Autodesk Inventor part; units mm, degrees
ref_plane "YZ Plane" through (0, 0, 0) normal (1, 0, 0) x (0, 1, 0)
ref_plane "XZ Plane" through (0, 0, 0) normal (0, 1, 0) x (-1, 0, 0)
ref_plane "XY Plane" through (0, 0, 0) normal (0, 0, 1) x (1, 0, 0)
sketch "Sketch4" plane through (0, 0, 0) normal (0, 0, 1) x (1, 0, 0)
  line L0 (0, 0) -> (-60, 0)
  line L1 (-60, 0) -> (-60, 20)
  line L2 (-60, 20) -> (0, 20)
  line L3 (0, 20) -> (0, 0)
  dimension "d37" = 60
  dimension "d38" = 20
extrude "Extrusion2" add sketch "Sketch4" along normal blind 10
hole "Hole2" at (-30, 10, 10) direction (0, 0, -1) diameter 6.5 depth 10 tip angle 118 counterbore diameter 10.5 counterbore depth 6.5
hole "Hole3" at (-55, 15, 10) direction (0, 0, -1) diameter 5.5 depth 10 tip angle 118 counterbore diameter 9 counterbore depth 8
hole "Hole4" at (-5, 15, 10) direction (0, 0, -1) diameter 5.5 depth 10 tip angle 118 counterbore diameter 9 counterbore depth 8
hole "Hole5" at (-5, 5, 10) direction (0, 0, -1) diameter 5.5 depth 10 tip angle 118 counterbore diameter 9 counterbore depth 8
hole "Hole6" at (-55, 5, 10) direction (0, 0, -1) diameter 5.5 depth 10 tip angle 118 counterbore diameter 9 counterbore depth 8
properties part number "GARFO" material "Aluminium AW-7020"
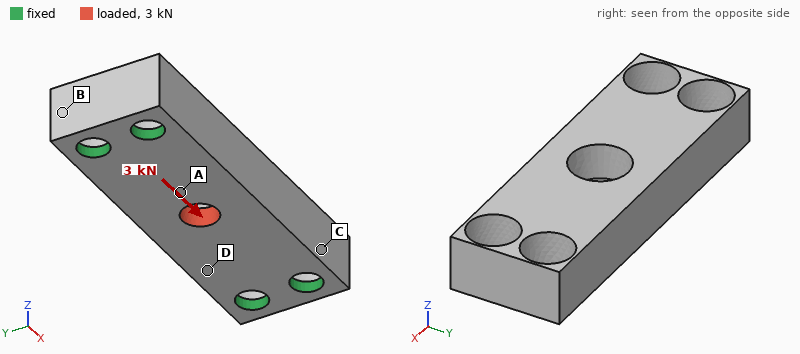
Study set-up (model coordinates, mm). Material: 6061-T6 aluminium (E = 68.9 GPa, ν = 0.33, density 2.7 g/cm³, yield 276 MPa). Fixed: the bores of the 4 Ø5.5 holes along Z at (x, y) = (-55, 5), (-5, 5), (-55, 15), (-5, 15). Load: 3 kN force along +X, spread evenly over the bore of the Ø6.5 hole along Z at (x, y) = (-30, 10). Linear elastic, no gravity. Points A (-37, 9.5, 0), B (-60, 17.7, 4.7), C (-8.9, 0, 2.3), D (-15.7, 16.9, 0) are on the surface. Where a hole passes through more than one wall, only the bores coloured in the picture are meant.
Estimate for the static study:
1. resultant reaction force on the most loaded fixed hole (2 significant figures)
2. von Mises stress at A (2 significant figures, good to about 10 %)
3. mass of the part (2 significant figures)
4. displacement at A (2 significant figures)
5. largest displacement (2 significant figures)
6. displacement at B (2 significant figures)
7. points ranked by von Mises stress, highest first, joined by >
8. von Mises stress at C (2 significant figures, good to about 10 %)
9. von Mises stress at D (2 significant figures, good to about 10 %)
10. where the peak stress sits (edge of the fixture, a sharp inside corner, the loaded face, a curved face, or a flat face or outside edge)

760 N
38 MPa
25 g
6.7 µm
8.9 µm
2.4 µm
A > D > C > B
13 MPa
23 MPa
the loaded face
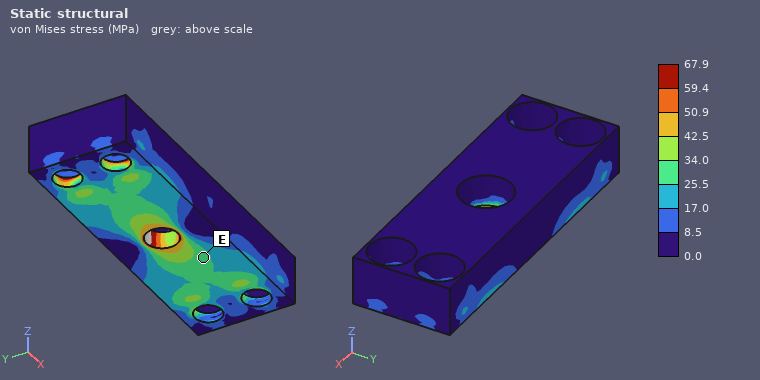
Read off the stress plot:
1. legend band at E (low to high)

25.5 to 34.0 MPa
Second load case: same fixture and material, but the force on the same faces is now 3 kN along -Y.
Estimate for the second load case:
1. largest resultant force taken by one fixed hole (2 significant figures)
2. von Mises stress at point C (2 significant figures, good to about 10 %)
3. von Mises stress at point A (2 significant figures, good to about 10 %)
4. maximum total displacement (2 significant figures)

1.0 kN
20 MPa
29 MPa
25 µm
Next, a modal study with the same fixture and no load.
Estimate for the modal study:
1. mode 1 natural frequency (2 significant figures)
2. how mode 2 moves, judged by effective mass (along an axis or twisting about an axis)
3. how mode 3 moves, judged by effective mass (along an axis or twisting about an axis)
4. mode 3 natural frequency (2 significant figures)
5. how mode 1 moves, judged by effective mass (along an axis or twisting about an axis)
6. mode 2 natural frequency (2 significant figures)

12 kHz
along Y
along Y
21 kHz
along Z
15 kHz
